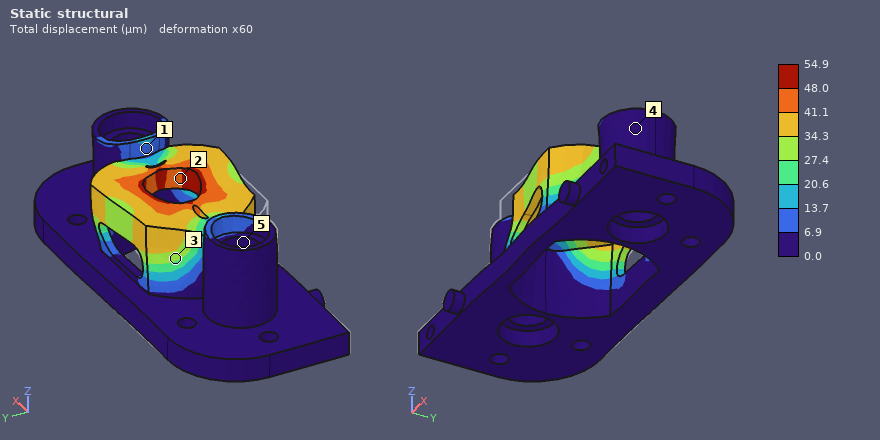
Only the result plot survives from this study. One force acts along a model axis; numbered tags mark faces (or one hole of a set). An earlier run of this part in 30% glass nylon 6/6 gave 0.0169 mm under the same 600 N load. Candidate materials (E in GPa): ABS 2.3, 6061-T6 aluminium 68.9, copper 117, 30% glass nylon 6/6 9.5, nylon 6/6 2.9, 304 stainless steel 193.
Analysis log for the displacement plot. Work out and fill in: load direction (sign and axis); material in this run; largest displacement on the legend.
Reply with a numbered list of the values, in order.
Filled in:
1. +X
2. nylon 6/6
3. 54.9 µm
